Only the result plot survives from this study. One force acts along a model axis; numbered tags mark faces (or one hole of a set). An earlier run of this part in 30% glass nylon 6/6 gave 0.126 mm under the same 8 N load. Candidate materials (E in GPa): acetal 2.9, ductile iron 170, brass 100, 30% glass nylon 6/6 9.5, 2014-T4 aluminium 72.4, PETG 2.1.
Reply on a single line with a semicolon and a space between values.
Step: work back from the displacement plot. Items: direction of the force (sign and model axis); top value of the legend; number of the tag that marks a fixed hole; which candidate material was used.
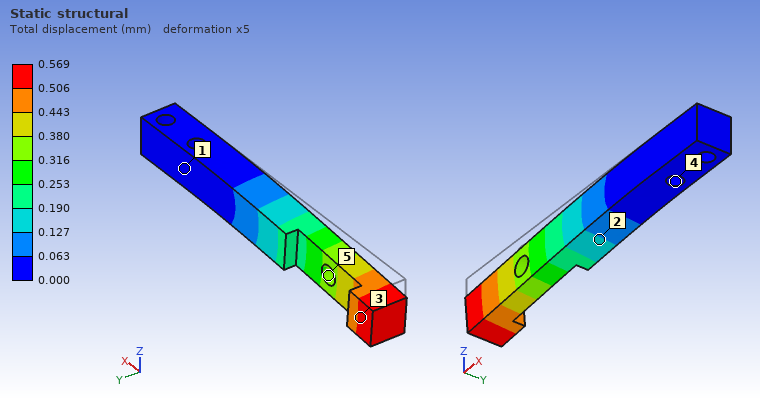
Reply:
-Z; 0.569 mm; 4; PETG
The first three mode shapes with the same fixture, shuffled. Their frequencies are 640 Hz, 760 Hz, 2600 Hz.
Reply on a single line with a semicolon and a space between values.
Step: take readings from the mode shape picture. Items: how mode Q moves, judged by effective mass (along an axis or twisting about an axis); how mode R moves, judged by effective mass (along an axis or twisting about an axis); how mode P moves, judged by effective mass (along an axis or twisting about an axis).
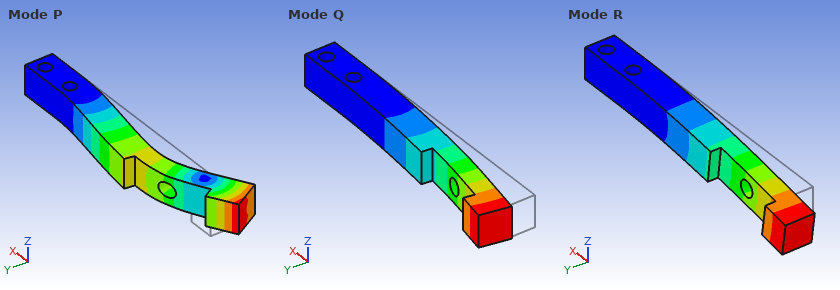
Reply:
along Y; along Z; along Y
